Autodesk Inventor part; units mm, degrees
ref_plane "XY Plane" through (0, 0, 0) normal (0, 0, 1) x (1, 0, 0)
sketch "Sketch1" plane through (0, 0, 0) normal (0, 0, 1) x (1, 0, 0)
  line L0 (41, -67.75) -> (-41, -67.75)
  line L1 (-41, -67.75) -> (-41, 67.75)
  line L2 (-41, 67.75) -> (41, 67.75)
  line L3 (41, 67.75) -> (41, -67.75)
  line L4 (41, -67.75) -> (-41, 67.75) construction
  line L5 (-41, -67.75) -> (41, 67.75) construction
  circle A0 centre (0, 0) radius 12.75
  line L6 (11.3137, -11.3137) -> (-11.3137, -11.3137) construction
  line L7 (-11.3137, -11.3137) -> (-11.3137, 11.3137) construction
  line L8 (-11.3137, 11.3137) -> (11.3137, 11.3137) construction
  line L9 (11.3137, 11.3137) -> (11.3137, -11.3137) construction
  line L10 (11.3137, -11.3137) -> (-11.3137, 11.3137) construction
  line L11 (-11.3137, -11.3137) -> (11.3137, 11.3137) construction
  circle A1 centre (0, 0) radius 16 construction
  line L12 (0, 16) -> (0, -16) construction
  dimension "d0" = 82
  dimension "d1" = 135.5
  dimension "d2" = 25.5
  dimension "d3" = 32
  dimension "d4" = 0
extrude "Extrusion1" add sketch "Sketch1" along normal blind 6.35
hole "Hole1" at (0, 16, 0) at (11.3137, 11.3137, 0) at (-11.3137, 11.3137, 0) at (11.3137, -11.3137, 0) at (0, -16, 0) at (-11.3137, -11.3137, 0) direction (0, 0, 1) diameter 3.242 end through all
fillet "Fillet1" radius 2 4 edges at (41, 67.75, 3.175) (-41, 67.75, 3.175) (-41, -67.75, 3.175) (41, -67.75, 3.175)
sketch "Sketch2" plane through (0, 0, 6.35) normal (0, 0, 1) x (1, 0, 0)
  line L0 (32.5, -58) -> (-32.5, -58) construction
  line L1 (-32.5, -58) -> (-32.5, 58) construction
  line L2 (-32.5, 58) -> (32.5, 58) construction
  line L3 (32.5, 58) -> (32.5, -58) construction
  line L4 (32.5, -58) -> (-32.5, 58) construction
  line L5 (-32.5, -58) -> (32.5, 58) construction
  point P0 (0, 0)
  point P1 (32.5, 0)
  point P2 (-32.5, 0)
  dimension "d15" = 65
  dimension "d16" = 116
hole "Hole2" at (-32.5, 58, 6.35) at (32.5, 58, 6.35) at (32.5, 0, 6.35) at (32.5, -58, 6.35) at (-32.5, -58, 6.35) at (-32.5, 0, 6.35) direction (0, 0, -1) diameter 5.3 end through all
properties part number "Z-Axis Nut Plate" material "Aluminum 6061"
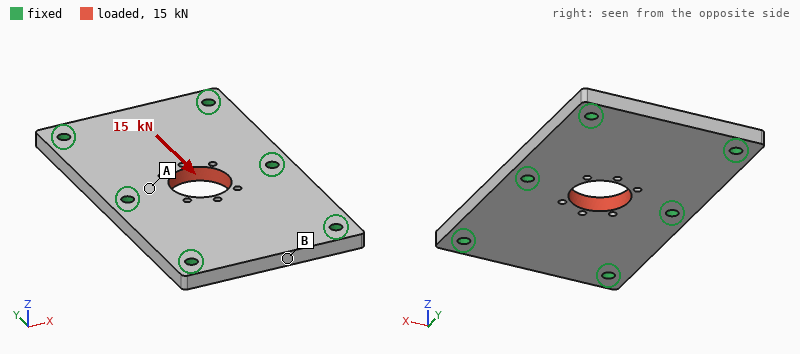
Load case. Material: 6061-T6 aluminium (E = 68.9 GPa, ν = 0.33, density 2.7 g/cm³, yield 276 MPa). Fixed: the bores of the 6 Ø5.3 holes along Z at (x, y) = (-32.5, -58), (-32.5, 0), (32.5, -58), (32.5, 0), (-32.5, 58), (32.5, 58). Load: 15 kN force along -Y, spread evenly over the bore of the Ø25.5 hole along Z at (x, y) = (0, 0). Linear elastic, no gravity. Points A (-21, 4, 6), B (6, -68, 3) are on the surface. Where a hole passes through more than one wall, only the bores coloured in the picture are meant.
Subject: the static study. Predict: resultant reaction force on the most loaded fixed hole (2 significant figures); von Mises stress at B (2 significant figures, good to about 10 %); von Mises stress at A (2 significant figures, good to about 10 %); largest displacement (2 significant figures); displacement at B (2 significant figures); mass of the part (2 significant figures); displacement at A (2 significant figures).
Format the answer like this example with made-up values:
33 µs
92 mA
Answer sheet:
3.6 kN
8.9 MPa
21 MPa
19 µm
6.7 µm
180 g
8.4 µm
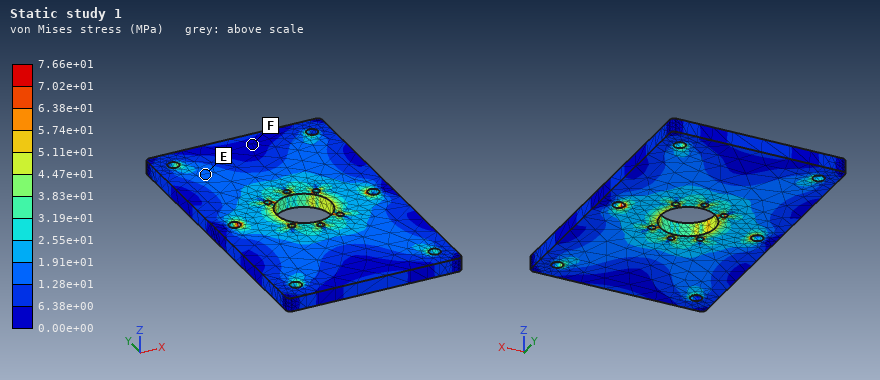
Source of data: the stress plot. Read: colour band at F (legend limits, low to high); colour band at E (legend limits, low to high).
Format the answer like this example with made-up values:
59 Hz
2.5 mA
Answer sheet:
0.00e+00 to 6.38e+00 MPa
1.28e+01 to 1.91e+01 MPa
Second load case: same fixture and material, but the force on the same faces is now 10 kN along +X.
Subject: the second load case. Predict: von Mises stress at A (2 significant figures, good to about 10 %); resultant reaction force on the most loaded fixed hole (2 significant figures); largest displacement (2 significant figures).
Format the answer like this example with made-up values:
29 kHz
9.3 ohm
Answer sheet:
27 MPa
3.6 kN
11 µm
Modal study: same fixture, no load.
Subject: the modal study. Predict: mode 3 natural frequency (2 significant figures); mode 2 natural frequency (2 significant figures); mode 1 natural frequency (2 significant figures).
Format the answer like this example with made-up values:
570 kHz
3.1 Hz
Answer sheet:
8800 Hz
5900 Hz
5700 Hz
